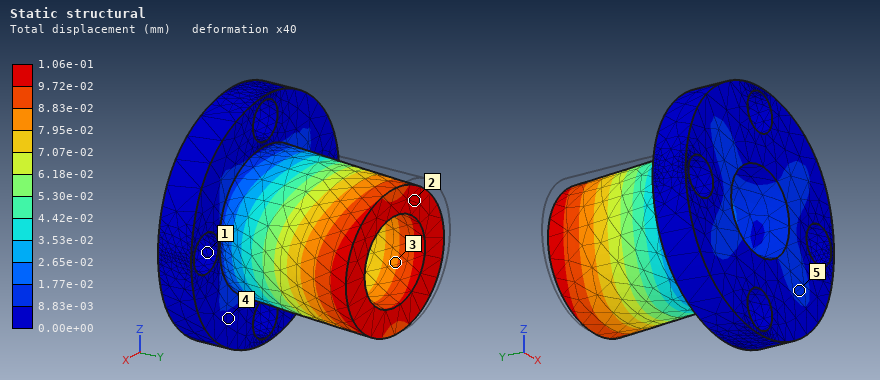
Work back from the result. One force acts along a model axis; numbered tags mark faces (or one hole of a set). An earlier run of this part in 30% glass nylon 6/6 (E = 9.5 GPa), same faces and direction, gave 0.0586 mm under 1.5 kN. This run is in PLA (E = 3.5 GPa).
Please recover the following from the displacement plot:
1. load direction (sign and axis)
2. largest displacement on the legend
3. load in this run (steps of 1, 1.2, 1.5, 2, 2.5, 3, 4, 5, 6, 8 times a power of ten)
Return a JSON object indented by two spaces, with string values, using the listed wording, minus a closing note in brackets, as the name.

{
  "load direction": "+X",
  "largest displacement on the legend": "1.06e-01 mm",
  "load in this run": "1 kN"
}
